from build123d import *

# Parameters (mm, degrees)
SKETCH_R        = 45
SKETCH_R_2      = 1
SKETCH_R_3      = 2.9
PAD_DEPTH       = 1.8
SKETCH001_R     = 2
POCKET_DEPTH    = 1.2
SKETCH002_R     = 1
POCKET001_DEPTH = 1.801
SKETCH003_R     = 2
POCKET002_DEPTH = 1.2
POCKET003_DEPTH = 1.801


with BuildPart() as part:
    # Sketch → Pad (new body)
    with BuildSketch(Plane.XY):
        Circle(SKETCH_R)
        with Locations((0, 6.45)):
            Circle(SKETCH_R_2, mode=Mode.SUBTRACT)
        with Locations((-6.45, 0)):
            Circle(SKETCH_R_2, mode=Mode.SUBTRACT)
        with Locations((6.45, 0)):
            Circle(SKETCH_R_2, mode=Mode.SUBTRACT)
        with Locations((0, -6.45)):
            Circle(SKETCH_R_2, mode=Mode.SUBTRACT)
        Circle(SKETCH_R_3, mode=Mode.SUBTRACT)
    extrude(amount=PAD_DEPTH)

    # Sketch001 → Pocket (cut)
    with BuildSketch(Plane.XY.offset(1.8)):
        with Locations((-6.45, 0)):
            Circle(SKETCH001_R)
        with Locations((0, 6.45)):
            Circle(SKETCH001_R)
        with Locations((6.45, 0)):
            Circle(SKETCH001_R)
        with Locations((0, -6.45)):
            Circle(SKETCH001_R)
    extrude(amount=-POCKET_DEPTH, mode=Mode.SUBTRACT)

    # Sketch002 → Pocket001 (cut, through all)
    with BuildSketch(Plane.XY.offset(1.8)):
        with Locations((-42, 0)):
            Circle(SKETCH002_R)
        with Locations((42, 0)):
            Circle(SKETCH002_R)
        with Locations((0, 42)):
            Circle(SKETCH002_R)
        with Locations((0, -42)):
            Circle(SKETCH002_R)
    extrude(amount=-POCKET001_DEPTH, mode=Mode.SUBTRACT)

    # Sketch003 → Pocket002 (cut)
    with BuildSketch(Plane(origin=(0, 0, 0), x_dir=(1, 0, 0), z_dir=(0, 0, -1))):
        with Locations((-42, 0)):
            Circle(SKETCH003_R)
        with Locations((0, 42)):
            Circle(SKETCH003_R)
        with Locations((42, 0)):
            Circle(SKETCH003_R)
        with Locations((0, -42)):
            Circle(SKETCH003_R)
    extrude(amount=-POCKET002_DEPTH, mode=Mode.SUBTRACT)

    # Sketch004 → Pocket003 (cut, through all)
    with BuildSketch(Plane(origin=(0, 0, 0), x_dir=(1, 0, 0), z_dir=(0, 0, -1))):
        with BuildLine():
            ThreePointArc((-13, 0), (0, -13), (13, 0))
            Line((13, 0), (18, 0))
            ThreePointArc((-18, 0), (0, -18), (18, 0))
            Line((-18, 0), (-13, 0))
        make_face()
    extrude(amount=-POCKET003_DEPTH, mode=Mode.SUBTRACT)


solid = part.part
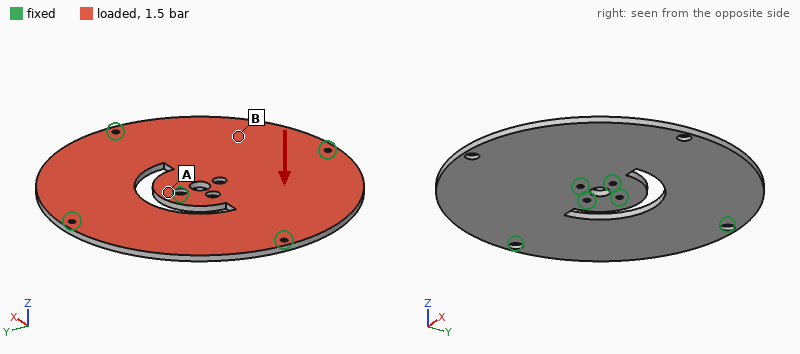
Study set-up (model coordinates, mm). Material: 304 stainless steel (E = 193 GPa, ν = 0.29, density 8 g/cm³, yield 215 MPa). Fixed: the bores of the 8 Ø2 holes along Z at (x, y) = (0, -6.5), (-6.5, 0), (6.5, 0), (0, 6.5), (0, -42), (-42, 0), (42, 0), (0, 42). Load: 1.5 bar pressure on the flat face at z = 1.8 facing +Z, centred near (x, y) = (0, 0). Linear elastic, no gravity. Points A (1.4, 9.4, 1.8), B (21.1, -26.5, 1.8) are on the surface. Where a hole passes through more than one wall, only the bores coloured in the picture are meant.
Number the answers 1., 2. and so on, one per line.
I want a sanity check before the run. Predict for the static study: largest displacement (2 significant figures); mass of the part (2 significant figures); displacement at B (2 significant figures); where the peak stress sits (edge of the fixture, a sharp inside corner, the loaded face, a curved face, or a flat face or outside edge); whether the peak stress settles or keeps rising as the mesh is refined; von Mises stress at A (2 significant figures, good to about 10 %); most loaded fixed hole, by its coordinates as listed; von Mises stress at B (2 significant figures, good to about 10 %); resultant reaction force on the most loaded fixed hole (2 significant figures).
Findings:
1. 84 µm
2. 87 g
3. 55 µm
4. edge of the fixture
5. keeps rising
6. 14 MPa
7. (0, 42)
8. 25 MPa
9. 350 N
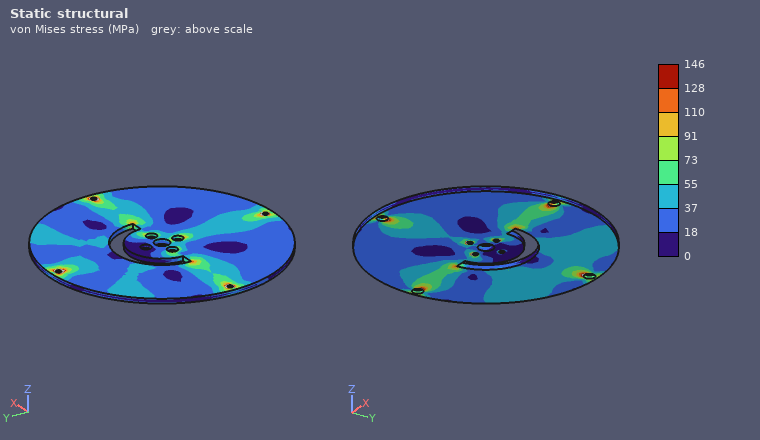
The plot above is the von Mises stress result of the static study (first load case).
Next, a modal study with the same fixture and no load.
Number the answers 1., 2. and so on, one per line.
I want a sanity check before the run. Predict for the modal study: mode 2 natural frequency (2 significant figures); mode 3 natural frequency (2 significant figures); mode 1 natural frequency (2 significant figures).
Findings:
1. 1900 Hz
2. 2000 Hz
3. 1600 Hz
